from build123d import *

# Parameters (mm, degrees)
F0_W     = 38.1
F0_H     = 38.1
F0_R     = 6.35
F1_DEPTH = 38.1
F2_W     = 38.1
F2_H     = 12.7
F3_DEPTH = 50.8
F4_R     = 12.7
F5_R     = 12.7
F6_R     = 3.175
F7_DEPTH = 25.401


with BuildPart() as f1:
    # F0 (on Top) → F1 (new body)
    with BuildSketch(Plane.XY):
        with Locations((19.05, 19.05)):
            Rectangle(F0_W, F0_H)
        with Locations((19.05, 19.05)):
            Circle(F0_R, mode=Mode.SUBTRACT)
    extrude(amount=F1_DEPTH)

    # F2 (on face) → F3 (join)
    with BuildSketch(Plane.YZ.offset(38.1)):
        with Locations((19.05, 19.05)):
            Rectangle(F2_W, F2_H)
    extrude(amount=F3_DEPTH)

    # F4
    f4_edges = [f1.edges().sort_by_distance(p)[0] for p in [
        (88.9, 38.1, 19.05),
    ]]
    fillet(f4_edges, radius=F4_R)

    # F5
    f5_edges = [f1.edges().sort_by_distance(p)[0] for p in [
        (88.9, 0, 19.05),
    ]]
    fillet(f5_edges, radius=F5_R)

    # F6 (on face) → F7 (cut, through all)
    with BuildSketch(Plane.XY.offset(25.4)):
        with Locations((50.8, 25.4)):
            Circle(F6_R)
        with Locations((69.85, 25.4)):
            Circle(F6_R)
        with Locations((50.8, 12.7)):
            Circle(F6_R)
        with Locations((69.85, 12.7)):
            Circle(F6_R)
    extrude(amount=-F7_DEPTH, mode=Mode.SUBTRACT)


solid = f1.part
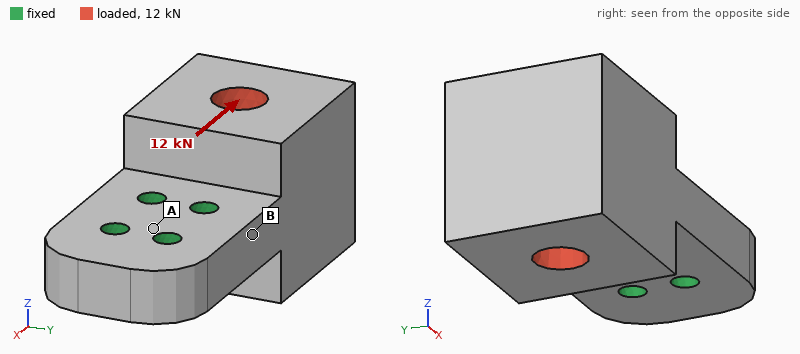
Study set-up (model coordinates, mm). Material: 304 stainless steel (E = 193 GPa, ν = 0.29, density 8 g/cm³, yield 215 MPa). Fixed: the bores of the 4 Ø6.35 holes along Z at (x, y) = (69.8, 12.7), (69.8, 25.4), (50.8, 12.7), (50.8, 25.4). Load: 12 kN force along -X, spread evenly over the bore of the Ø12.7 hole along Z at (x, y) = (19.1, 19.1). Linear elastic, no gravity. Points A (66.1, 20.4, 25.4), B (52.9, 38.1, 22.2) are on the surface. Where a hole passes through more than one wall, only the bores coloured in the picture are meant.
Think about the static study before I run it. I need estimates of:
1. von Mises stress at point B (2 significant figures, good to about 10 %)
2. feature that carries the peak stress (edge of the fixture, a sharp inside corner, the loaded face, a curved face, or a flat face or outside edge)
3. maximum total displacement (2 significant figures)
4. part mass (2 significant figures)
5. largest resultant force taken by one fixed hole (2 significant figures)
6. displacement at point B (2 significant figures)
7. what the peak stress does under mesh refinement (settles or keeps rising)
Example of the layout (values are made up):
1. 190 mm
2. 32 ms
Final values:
1. 14 MPa
2. edge of the fixture
3. 4.3 µm
4. 580 g
5. 5.4 kN
6. 0.88 µm
7. keeps rising
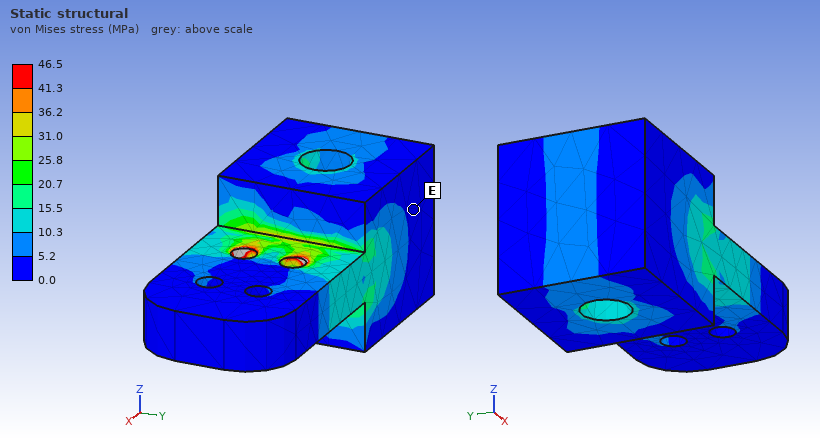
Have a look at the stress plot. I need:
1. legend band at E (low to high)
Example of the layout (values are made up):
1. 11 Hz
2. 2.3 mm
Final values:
1. 0.0 to 5.2 MPa
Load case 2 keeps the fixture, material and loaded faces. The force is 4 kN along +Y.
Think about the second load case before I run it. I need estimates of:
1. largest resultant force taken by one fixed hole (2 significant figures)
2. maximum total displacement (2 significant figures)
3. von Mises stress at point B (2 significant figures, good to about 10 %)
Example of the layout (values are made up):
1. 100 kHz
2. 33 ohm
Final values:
1. 5.1 kN
2. 14 µm
3. 29 MPa
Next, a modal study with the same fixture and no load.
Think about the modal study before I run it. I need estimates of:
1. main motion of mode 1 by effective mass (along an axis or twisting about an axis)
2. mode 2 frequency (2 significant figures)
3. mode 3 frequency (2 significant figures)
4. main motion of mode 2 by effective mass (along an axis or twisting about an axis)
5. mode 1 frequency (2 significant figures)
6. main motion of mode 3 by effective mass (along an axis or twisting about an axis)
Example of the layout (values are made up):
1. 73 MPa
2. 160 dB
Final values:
1. along Z
2. 4800 Hz
3. 6300 Hz
4. along Y
5. 2400 Hz
6. twisting about X
